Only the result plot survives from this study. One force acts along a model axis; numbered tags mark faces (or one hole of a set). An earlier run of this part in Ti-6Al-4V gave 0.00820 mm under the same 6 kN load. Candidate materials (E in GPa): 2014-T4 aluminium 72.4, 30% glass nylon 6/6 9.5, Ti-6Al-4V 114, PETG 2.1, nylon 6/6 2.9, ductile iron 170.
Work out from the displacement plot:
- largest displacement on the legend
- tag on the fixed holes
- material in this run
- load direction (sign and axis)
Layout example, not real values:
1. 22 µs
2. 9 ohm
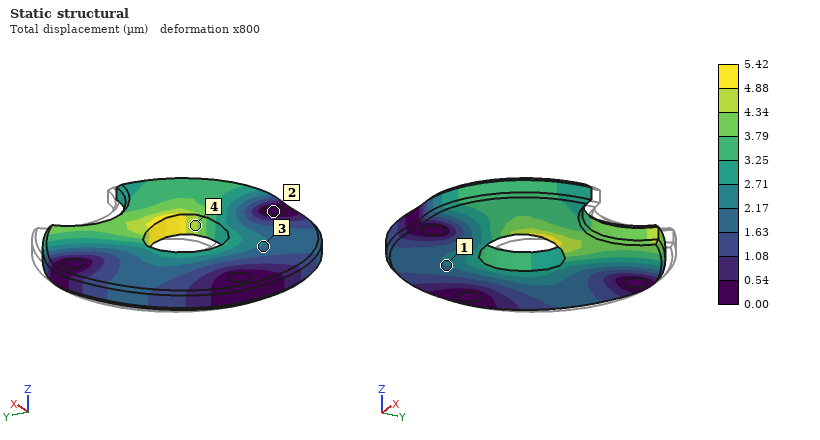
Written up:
1. 5.42 µm
2. 2
3. ductile iron
4. -Y
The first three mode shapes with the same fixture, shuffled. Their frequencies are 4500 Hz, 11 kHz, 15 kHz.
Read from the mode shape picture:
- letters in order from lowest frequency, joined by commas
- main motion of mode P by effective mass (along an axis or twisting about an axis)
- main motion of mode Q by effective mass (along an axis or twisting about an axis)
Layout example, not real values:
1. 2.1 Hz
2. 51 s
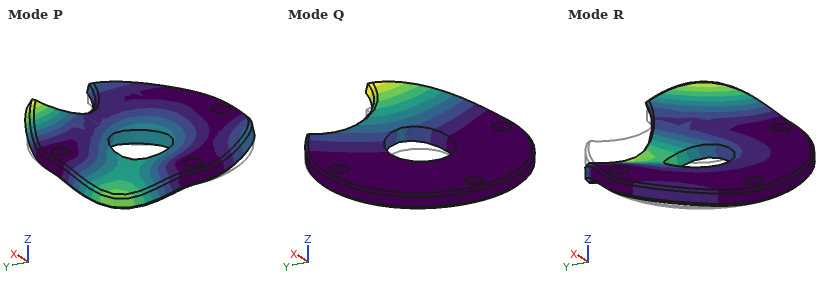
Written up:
1. Q, R, P
2. along Z
3. along Z
